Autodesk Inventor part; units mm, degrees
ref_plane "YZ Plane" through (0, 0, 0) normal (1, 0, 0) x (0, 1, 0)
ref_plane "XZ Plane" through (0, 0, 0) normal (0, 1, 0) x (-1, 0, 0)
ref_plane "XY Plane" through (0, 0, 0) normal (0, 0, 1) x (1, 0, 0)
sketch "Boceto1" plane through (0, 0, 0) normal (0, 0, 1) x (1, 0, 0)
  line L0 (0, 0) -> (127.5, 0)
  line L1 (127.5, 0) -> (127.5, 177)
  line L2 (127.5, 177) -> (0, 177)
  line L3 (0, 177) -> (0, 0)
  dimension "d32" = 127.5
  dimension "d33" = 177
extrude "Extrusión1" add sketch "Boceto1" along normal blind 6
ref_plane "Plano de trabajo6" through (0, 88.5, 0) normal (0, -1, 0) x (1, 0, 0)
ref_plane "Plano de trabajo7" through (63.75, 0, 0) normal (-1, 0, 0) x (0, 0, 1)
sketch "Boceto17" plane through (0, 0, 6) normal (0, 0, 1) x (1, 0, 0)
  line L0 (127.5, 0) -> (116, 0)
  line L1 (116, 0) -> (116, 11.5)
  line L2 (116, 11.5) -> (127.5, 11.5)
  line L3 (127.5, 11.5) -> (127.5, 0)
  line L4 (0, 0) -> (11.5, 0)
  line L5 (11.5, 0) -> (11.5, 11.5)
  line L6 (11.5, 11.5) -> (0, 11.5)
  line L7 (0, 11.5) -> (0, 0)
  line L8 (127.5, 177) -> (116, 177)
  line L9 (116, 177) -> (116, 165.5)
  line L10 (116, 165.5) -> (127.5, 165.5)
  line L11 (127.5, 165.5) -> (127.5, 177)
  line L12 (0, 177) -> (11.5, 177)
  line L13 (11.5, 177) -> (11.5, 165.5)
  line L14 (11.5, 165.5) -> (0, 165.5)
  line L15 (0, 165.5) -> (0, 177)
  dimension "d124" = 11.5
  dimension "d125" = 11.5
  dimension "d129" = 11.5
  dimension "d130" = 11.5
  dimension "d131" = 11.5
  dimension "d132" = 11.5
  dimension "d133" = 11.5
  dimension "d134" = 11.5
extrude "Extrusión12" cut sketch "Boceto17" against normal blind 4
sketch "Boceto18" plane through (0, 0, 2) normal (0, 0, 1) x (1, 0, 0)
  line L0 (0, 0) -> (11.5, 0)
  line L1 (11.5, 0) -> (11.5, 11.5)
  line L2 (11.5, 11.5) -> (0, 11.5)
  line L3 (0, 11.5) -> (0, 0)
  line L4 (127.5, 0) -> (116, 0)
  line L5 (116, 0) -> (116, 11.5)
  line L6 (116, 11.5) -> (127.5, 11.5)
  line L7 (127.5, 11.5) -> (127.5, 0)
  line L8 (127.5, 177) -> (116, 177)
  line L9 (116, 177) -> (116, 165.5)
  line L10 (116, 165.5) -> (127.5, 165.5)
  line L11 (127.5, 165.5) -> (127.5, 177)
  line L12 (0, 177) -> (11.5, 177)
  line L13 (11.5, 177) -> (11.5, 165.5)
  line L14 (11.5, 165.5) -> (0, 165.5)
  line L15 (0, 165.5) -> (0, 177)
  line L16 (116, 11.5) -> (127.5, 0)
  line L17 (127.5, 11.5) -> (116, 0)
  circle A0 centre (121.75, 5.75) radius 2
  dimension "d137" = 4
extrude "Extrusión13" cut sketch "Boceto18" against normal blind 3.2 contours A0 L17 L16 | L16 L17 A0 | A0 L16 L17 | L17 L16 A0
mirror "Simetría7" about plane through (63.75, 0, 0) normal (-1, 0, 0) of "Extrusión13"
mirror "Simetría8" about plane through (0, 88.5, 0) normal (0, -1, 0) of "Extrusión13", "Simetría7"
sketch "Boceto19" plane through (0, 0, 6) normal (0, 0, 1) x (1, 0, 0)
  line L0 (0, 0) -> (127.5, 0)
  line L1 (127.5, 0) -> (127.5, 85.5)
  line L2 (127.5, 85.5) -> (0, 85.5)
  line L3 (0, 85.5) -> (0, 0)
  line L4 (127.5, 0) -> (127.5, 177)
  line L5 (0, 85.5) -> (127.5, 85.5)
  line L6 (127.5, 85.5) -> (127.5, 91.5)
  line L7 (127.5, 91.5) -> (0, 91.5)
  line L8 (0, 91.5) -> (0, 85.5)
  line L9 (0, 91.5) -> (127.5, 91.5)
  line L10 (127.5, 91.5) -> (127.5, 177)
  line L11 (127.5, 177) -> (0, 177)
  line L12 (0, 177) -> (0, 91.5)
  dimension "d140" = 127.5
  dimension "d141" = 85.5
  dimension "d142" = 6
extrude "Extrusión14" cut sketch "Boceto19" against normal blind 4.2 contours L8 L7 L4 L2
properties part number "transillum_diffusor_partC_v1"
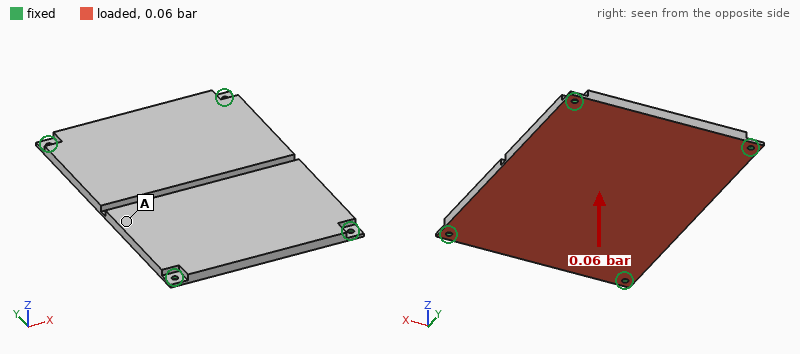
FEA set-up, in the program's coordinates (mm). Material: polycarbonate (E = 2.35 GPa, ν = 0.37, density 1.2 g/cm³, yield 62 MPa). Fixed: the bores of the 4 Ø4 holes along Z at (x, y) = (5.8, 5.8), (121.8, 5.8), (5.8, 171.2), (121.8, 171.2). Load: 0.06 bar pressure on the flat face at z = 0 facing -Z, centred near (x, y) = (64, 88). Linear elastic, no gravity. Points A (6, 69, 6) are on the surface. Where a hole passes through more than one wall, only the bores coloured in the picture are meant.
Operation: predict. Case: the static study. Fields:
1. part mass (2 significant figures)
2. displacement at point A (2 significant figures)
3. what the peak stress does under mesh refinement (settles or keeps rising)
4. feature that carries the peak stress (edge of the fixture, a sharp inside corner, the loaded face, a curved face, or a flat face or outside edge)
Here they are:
160 g
2.0 mm
keeps rising
edge of the fixture
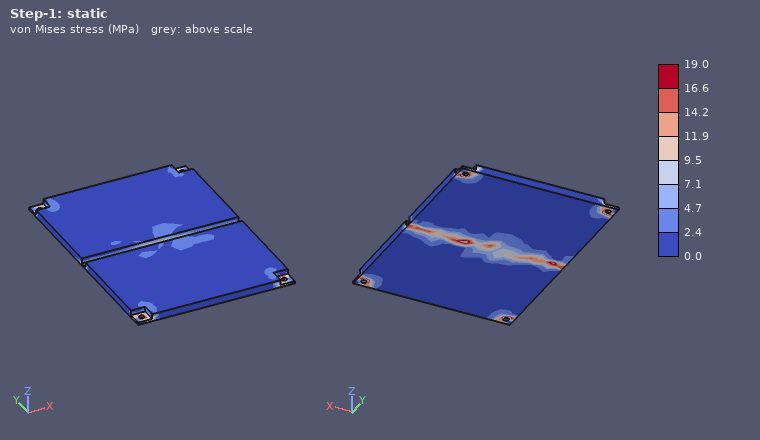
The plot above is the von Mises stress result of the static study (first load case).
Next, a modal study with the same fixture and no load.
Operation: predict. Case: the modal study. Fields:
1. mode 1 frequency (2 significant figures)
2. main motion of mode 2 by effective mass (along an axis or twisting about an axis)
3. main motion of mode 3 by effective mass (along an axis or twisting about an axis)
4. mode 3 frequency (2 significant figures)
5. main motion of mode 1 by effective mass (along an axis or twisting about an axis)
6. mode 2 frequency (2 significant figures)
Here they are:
110 Hz
twisting about Y
twisting about X
430 Hz
along Z
290 Hz
